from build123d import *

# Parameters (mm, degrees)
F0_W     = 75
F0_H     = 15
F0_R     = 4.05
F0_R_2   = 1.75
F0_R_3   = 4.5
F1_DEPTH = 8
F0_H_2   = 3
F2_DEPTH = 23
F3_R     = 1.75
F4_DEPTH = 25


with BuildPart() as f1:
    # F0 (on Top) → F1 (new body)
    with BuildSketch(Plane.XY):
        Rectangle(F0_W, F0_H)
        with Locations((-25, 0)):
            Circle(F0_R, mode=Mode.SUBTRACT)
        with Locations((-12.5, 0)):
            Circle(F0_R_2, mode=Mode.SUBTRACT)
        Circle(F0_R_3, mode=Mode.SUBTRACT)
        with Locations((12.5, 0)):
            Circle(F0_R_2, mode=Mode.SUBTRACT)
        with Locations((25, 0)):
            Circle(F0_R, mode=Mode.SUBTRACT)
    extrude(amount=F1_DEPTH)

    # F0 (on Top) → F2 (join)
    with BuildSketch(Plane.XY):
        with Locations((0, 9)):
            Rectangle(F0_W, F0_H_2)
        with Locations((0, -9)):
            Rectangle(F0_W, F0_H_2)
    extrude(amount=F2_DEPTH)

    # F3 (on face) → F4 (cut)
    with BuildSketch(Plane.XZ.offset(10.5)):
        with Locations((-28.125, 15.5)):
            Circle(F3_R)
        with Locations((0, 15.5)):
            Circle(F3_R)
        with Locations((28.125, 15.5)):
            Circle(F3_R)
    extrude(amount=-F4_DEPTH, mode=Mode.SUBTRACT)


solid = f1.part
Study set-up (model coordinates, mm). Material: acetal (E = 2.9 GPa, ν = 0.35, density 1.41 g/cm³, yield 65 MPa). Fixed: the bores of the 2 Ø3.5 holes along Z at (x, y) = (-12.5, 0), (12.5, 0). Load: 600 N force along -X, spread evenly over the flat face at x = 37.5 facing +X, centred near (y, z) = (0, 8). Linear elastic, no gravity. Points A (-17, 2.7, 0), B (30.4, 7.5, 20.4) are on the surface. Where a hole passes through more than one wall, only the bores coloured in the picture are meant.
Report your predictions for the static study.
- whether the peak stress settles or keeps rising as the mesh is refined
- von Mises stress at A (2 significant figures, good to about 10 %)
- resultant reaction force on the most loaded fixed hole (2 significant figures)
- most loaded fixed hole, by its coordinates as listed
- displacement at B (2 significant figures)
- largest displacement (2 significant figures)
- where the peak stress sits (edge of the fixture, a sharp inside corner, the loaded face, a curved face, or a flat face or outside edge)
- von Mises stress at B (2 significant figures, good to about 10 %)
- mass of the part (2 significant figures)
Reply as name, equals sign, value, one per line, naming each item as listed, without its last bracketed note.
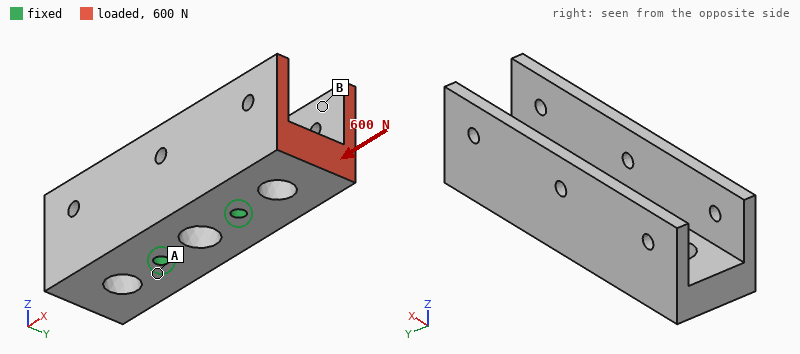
whether the peak stress settles or keeps rising as the mesh is refined = keeps rising
von Mises stress at A = 1.3 MPa
resultant reaction force on the most loaded fixed hole = 430 N
most loaded fixed hole, by its coordinates as listed = (12.5, 0)
displacement at B = 53 µm
largest displacement = 64 µm
where the peak stress sits = edge of the fixture
von Mises stress at B = 2.9 MPa
mass of the part = 25 g
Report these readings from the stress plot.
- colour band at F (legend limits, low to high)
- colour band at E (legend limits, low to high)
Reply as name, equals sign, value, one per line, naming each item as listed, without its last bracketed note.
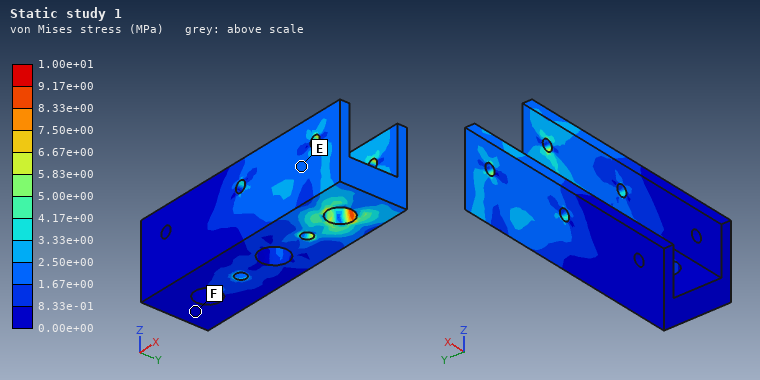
colour band at F = 0.00e+00 to 8.33e-01 MPa
colour band at E = 1.67e+00 to 2.50e+00 MPa
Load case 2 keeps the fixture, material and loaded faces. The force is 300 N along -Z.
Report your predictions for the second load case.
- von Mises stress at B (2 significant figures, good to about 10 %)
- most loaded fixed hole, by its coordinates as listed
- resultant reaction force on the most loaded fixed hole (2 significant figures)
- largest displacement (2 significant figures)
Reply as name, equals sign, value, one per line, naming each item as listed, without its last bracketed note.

von Mises stress at B = 2.7 MPa
most loaded fixed hole, by its coordinates as listed = (12.5, 0)
resultant reaction force on the most loaded fixed hole = 510 N
largest displacement = 0.26 mm
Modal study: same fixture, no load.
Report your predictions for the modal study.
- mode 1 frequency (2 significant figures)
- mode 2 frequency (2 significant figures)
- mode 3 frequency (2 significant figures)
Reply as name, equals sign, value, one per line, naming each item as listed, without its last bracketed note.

mode 1 frequency = 2000 Hz
mode 2 frequency = 2000 Hz
mode 3 frequency = 2400 Hz
